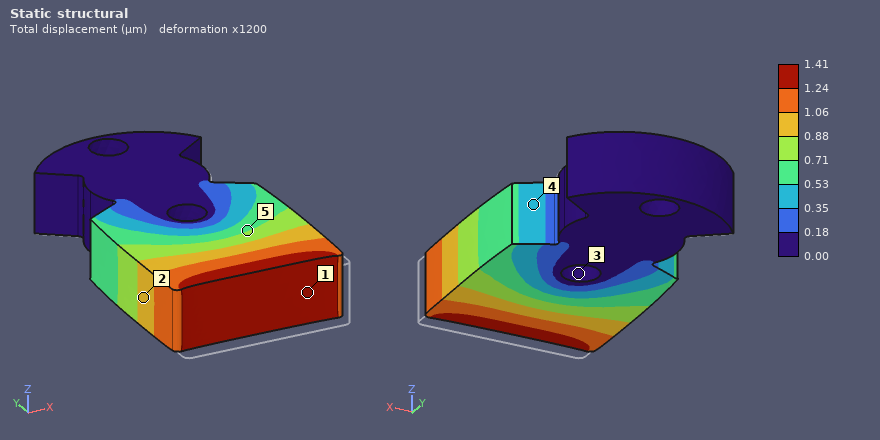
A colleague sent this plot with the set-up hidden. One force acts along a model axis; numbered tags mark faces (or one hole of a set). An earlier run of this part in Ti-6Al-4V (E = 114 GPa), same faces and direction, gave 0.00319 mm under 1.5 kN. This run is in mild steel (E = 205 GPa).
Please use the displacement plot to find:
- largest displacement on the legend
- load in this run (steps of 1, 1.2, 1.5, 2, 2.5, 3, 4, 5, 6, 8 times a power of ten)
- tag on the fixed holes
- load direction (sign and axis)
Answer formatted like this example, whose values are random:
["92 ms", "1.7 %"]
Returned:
["1.41 µm", "1.2 kN", "3", "+Y"]
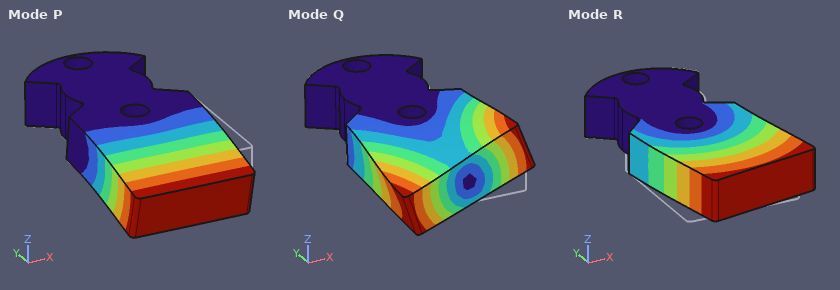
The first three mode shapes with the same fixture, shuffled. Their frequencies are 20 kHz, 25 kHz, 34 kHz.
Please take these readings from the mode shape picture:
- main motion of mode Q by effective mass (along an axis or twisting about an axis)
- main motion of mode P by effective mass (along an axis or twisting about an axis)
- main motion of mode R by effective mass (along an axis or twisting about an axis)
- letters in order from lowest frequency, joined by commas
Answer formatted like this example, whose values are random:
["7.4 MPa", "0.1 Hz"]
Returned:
["twisting about Y", "along Z", "along X", "P, R, Q"]
